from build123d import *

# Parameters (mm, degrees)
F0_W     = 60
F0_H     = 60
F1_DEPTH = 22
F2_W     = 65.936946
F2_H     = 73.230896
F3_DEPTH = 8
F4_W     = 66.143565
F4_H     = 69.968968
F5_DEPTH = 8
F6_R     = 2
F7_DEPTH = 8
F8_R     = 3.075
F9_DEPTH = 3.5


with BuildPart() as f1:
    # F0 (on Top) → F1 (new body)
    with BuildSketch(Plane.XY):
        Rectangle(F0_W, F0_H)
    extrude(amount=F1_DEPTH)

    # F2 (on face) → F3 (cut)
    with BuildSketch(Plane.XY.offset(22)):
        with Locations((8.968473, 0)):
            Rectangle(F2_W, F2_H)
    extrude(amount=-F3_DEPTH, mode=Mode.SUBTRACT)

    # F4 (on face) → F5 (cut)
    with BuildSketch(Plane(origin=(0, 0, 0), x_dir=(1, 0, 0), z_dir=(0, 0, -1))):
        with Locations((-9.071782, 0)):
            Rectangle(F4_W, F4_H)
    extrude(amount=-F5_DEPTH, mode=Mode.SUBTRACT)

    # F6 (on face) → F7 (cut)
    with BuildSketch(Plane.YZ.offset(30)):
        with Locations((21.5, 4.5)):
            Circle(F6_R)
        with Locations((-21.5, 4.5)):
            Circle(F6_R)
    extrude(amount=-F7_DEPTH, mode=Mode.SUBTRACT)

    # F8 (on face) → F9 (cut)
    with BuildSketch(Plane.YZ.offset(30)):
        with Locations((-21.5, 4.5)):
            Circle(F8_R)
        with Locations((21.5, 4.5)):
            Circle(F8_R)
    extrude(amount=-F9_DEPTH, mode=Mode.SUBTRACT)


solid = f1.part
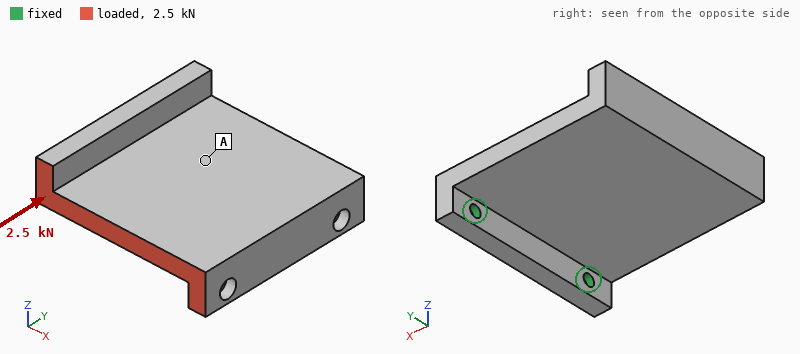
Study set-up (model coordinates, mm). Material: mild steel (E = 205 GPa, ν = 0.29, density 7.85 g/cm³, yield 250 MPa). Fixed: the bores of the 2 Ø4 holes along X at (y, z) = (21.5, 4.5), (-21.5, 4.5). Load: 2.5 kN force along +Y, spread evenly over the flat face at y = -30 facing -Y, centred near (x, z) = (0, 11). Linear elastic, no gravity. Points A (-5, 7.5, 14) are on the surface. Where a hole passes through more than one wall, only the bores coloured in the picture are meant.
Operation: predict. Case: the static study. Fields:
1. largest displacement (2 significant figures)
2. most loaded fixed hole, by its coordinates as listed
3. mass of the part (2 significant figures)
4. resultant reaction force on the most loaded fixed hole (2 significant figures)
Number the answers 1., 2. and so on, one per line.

1. 24 µm
2. (-21.5, 4.5)
3. 210 g
4. 2.1 kN
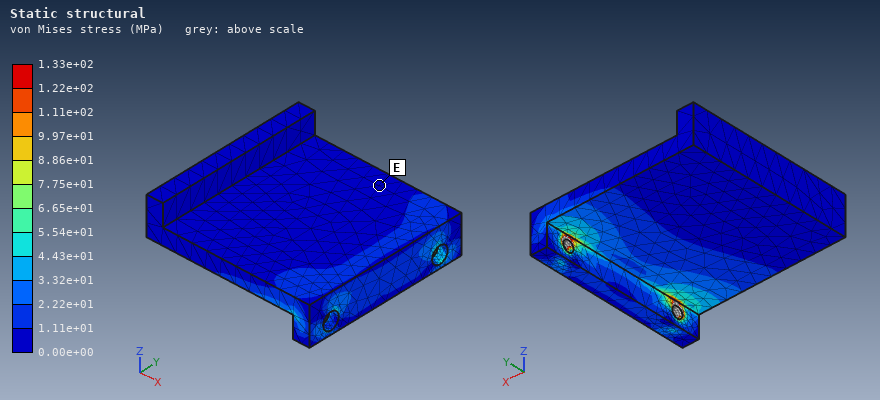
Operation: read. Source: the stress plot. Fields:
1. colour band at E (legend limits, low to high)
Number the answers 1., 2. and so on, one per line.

1. 0.00e+00 to 1.11e+01 MPa
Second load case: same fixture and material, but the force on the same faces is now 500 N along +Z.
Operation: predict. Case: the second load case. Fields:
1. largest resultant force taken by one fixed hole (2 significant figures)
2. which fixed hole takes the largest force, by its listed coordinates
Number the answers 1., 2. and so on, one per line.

1. 590 N
2. (-21.5, 4.5)
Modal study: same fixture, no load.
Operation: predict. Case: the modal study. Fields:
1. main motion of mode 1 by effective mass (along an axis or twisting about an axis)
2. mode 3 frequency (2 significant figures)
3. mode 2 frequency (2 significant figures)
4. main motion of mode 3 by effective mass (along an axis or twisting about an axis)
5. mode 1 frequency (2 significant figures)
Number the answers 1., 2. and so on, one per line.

1. along Z
2. 4200 Hz
3. 2800 Hz
4. along Y
5. 740 Hz
